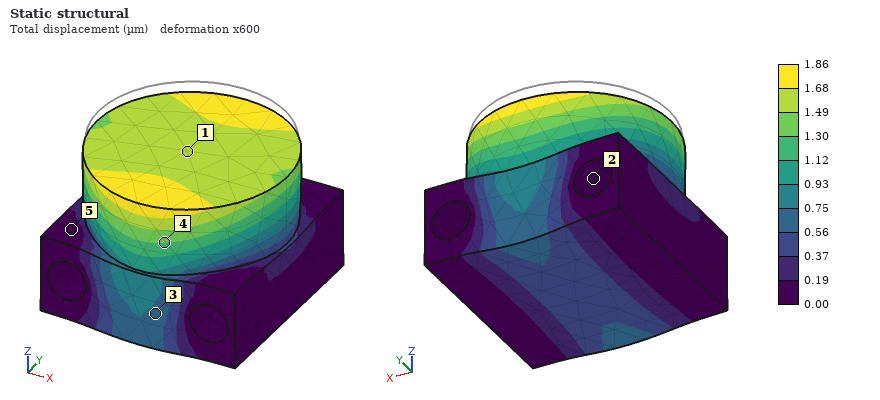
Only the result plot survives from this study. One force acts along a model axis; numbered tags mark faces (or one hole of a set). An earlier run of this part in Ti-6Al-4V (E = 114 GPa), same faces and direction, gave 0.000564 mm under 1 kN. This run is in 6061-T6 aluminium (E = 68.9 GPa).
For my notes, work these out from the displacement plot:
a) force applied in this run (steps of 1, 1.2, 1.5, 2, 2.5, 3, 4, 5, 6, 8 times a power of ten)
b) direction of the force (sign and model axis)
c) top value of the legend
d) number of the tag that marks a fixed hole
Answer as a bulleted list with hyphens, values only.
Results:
- 2 kN
- -Z
- 1.86 µm
- 2
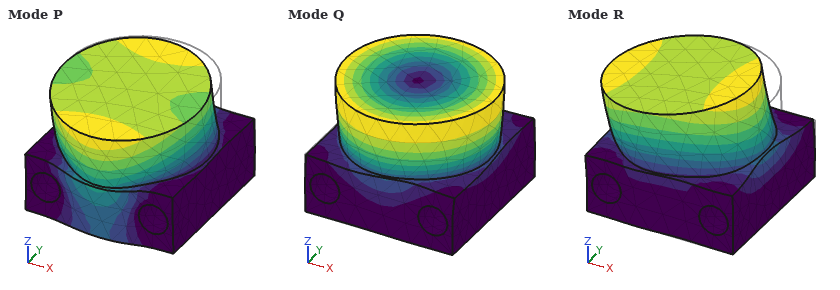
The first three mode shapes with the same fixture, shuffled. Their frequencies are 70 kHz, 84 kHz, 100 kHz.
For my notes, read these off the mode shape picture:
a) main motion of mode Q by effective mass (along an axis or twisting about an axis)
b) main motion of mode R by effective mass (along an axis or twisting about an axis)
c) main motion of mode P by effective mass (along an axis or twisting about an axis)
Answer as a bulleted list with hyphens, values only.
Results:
- twisting about Z
- along X
- along Y
